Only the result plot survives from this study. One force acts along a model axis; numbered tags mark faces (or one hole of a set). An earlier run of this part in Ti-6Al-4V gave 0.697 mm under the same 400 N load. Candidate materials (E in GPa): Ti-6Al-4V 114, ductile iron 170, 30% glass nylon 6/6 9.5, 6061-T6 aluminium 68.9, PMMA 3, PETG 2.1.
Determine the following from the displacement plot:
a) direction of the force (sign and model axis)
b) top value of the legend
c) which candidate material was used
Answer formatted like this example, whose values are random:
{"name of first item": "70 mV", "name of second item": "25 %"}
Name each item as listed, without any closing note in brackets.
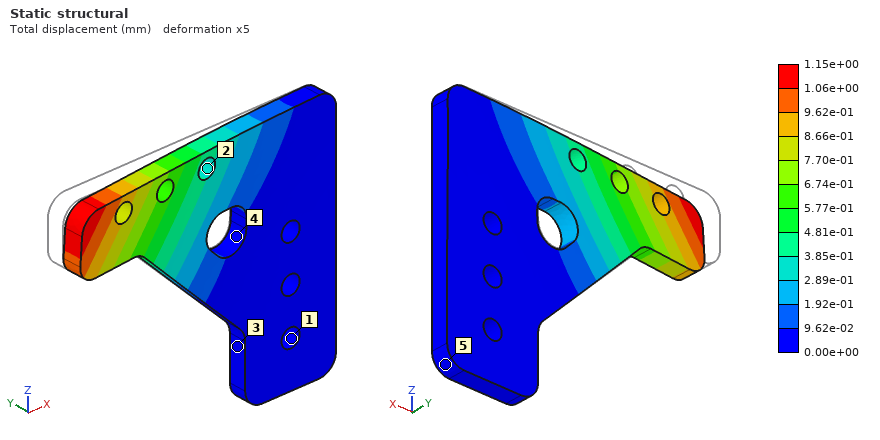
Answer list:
{"direction of the force": "-Y", "top value of the legend": "1.15e+00 mm", "which candidate material was used": "6061-T6 aluminium"}
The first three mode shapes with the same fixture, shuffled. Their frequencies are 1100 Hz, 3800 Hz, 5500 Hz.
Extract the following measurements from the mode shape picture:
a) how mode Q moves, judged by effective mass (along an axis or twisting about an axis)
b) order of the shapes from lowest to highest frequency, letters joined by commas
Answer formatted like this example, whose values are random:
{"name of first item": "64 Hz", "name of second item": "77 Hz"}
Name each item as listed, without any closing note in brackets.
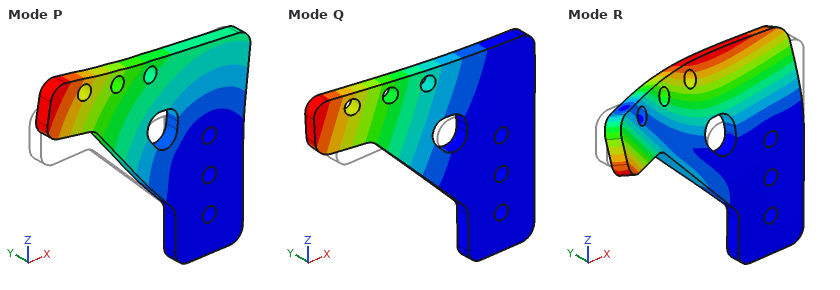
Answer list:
{"how mode Q moves, judged by effective mass": "along Y", "order of the shapes from lowest to highest frequency, letters joined by commas": "Q, R, P"}
